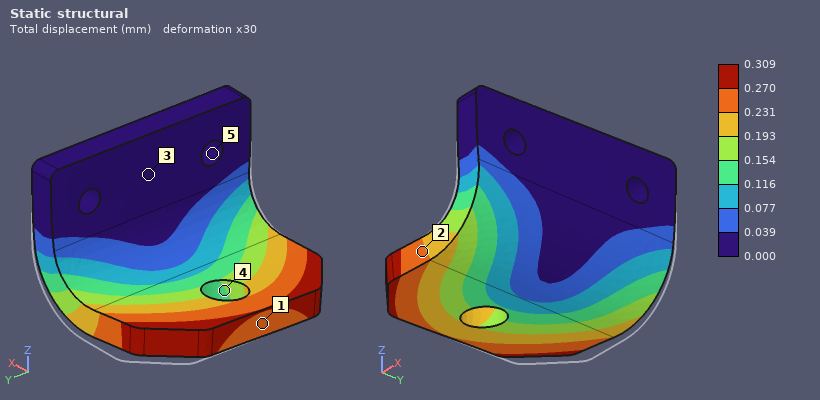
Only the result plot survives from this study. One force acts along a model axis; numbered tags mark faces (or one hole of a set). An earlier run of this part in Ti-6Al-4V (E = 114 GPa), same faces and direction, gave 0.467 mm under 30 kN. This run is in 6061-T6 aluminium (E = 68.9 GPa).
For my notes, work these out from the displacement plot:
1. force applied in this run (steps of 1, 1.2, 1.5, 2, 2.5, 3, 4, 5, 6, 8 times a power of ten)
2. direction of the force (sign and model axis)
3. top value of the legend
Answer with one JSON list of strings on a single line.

["12 kN", "-Y", "0.309 mm"]
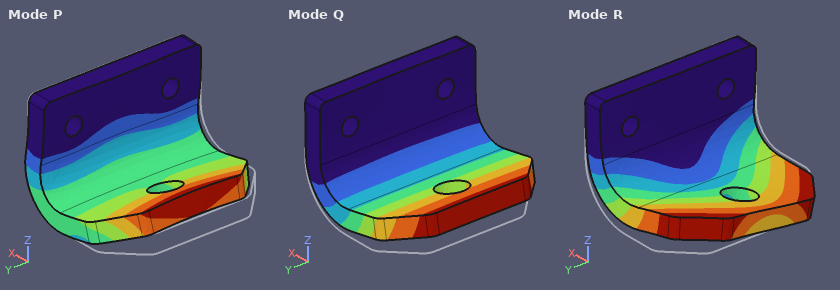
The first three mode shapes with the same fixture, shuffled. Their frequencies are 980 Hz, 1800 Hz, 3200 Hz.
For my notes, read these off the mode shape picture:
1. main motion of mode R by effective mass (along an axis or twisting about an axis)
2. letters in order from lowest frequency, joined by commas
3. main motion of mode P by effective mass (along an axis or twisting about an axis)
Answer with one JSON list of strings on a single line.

["along Y", "Q, R, P", "along X"]
